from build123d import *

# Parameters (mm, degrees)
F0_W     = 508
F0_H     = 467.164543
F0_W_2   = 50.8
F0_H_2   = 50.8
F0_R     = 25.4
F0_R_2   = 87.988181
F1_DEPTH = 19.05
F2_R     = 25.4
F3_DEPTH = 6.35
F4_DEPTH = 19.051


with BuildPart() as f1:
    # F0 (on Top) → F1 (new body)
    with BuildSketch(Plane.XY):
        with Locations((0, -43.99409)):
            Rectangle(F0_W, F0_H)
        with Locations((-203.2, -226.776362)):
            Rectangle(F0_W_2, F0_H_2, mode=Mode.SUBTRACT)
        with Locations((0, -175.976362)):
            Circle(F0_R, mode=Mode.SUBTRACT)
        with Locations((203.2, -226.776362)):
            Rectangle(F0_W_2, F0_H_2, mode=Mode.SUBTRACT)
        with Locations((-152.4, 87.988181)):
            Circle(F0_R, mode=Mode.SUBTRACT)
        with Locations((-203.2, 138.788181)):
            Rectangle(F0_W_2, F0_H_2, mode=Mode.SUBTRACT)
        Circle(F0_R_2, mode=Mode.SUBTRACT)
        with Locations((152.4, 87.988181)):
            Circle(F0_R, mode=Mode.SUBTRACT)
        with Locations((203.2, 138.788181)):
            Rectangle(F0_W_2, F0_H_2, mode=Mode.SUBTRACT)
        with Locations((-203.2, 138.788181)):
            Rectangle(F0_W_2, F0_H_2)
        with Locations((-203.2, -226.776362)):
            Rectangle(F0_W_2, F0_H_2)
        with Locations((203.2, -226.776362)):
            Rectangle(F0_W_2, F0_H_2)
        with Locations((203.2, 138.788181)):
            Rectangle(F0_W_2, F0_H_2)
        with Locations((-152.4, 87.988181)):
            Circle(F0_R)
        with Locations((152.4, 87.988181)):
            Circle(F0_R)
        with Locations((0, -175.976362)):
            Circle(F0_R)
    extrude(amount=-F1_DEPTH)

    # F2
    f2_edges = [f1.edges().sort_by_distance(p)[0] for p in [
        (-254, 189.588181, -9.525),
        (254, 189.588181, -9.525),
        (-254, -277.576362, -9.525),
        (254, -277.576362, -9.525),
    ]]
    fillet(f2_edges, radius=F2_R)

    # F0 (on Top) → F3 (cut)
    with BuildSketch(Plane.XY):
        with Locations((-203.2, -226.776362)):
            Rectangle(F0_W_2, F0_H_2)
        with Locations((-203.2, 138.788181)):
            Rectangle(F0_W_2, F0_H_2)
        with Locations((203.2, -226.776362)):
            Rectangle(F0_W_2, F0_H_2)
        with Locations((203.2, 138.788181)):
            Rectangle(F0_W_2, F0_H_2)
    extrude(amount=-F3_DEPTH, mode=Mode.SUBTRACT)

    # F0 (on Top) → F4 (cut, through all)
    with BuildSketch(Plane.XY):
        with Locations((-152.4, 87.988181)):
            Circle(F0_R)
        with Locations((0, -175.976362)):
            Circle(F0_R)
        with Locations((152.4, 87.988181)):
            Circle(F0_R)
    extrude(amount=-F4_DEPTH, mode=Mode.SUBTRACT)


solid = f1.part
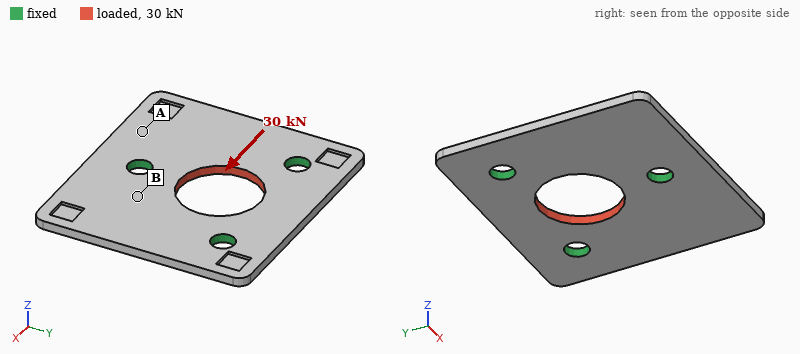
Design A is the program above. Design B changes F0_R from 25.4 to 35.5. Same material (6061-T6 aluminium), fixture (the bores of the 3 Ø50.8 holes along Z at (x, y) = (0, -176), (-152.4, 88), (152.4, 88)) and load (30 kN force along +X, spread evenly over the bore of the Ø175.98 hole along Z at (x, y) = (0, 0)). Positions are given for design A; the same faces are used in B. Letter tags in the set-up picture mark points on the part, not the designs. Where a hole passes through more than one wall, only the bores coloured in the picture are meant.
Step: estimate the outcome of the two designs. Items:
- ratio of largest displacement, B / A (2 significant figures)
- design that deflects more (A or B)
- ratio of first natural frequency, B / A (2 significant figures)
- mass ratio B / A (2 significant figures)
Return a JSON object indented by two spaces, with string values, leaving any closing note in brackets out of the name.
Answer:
{
  "ratio of largest displacement, B / A": "0.87",
  "design that deflects more": "A",
  "ratio of first natural frequency, B / A": "1.1",
  "mass ratio B / A": "0.97"
}
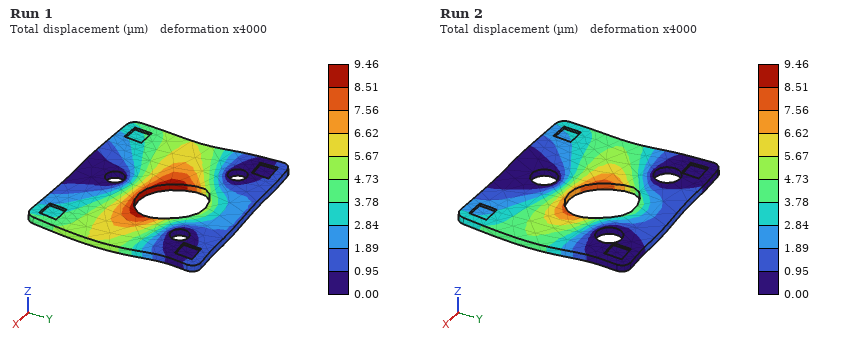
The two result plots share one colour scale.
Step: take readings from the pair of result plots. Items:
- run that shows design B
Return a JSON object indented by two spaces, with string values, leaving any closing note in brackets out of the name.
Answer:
{
  "run that shows design B": "Run 2"
}
